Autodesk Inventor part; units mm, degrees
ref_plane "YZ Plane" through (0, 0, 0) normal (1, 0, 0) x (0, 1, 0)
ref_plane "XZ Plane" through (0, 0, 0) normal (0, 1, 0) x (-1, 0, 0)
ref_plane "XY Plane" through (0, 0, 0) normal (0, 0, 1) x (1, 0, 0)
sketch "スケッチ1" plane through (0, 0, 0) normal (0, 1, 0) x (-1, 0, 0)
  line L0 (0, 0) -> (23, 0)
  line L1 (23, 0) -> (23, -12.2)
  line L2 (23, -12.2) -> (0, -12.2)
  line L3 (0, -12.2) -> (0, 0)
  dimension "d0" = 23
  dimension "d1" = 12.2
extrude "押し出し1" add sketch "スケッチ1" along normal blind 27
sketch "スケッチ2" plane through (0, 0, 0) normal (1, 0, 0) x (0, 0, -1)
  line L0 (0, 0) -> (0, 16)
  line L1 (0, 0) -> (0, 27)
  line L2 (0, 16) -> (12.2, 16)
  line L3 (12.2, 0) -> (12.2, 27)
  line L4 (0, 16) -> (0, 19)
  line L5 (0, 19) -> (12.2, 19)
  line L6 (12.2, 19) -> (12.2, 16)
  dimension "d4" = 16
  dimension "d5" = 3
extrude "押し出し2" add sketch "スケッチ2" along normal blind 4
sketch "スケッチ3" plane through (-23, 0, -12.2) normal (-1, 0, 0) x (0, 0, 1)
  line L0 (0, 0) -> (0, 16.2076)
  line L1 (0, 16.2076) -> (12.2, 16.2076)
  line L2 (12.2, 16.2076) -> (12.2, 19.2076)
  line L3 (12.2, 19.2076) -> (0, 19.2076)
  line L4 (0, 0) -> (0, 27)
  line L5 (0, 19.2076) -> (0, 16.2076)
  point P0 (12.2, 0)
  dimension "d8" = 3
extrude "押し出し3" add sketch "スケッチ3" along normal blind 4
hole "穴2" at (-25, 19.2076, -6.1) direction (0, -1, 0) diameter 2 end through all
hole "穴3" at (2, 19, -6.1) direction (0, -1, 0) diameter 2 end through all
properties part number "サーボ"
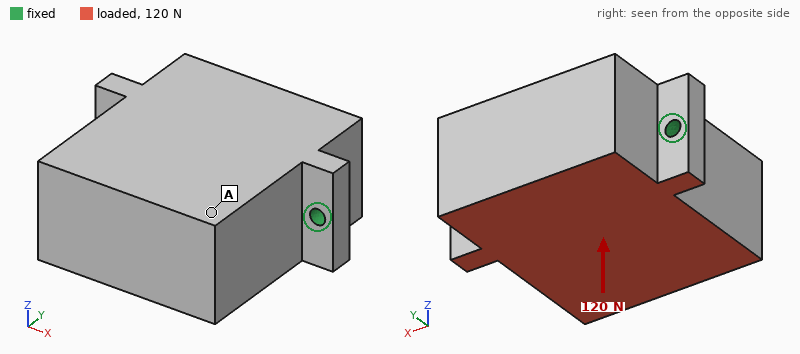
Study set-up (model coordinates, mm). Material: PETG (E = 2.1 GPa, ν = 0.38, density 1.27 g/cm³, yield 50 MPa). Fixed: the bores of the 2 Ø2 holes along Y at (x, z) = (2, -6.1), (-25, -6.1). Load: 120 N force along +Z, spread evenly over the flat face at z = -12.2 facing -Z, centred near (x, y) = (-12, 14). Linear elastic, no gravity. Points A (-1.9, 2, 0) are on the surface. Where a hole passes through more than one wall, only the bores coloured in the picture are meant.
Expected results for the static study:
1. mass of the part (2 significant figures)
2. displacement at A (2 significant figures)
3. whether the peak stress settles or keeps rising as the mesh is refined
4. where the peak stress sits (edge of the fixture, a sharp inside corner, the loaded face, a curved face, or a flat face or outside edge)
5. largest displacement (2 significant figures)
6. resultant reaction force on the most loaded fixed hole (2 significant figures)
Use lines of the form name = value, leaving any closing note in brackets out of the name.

mass of the part = 10.0 g
displacement at A = 0.19 mm
whether the peak stress settles or keeps rising as the mesh is refined = keeps rising
where the peak stress sits = edge of the fixture
largest displacement = 0.22 mm
resultant reaction force on the most loaded fixed hole = 60 N
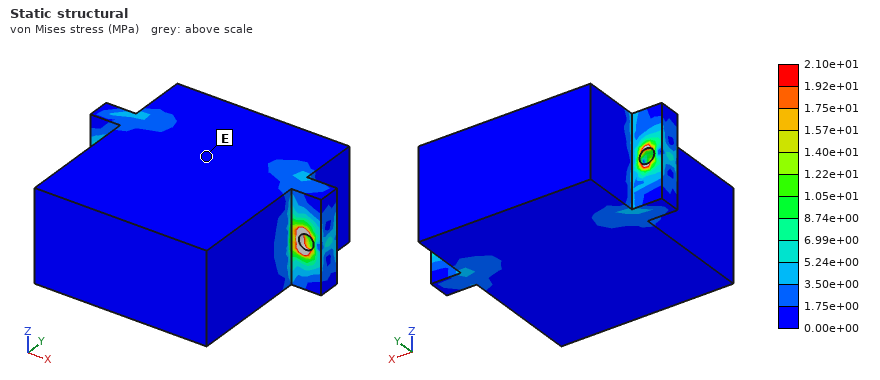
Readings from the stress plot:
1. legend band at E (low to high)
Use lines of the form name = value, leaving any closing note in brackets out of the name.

legend band at E = 0.00e+00 to 1.75e+00 MPa
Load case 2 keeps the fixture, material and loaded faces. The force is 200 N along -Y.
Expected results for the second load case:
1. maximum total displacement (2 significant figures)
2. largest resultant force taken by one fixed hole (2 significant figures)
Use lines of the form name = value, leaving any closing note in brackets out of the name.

maximum total displacement = 0.50 mm
largest resultant force taken by one fixed hole = 100 N
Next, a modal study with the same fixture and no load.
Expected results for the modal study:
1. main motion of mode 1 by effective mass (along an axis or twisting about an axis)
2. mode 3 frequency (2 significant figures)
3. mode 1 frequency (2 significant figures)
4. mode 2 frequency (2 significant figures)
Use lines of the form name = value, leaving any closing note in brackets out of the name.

main motion of mode 1 by effective mass = along Z
mode 3 frequency = 4600 Hz
mode 1 frequency = 1100 Hz
mode 2 frequency = 4500 Hz
